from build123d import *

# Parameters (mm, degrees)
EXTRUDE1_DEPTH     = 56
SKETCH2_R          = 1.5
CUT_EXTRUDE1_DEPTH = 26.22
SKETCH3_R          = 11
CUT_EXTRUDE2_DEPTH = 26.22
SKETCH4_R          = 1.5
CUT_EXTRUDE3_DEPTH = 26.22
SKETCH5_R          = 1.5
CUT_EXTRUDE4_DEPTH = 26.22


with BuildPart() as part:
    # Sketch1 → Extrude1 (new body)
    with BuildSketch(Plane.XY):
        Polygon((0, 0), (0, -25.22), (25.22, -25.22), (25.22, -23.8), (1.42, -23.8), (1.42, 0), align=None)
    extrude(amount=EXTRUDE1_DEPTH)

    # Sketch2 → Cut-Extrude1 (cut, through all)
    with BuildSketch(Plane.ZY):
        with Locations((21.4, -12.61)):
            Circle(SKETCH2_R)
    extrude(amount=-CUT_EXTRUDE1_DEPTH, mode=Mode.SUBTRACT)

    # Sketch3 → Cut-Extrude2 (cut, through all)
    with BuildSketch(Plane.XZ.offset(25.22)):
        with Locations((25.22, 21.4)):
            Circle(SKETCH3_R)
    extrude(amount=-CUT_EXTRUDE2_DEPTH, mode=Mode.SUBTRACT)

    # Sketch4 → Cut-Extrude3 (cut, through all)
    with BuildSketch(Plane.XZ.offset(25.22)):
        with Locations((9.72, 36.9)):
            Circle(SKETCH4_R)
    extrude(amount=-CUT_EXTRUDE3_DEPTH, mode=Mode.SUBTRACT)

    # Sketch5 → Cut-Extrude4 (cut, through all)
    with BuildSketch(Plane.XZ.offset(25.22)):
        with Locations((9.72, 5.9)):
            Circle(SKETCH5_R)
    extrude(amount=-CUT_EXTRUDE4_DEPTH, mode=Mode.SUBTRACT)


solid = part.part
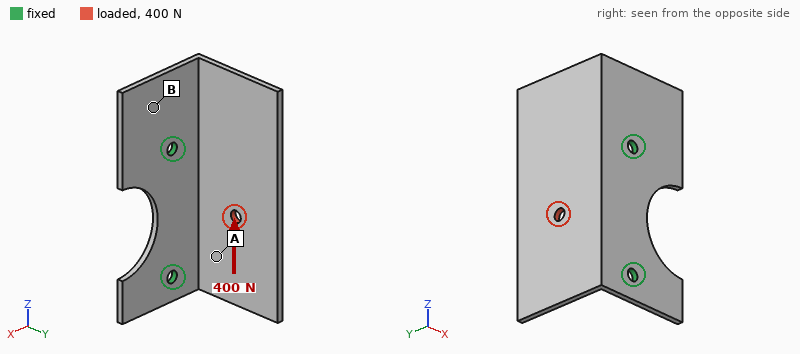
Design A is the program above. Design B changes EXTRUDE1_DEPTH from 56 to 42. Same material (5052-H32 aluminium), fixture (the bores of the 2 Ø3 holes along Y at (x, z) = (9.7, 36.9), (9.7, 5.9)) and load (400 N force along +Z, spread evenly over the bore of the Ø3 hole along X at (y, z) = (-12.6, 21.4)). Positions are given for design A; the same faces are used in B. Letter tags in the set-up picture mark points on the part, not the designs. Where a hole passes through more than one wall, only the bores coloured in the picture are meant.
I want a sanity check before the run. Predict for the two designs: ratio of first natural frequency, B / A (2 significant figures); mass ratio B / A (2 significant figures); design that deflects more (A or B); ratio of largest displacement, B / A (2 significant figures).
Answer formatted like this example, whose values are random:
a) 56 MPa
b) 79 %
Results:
a) 1.0
b) 0.73
c) A
d) 0.88
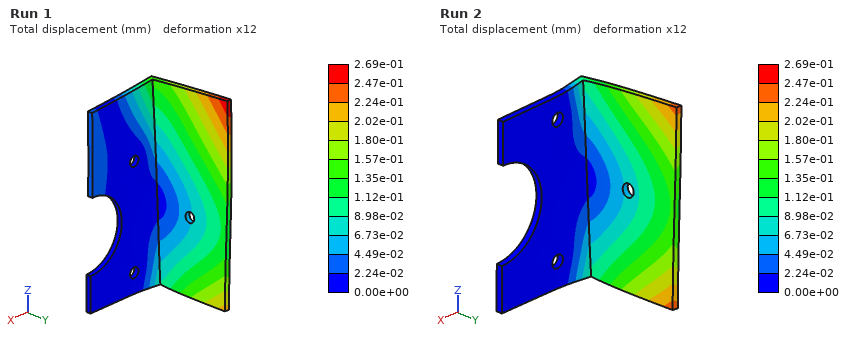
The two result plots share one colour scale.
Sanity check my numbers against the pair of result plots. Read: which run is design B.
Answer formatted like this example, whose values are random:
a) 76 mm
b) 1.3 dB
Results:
a) Run 2
